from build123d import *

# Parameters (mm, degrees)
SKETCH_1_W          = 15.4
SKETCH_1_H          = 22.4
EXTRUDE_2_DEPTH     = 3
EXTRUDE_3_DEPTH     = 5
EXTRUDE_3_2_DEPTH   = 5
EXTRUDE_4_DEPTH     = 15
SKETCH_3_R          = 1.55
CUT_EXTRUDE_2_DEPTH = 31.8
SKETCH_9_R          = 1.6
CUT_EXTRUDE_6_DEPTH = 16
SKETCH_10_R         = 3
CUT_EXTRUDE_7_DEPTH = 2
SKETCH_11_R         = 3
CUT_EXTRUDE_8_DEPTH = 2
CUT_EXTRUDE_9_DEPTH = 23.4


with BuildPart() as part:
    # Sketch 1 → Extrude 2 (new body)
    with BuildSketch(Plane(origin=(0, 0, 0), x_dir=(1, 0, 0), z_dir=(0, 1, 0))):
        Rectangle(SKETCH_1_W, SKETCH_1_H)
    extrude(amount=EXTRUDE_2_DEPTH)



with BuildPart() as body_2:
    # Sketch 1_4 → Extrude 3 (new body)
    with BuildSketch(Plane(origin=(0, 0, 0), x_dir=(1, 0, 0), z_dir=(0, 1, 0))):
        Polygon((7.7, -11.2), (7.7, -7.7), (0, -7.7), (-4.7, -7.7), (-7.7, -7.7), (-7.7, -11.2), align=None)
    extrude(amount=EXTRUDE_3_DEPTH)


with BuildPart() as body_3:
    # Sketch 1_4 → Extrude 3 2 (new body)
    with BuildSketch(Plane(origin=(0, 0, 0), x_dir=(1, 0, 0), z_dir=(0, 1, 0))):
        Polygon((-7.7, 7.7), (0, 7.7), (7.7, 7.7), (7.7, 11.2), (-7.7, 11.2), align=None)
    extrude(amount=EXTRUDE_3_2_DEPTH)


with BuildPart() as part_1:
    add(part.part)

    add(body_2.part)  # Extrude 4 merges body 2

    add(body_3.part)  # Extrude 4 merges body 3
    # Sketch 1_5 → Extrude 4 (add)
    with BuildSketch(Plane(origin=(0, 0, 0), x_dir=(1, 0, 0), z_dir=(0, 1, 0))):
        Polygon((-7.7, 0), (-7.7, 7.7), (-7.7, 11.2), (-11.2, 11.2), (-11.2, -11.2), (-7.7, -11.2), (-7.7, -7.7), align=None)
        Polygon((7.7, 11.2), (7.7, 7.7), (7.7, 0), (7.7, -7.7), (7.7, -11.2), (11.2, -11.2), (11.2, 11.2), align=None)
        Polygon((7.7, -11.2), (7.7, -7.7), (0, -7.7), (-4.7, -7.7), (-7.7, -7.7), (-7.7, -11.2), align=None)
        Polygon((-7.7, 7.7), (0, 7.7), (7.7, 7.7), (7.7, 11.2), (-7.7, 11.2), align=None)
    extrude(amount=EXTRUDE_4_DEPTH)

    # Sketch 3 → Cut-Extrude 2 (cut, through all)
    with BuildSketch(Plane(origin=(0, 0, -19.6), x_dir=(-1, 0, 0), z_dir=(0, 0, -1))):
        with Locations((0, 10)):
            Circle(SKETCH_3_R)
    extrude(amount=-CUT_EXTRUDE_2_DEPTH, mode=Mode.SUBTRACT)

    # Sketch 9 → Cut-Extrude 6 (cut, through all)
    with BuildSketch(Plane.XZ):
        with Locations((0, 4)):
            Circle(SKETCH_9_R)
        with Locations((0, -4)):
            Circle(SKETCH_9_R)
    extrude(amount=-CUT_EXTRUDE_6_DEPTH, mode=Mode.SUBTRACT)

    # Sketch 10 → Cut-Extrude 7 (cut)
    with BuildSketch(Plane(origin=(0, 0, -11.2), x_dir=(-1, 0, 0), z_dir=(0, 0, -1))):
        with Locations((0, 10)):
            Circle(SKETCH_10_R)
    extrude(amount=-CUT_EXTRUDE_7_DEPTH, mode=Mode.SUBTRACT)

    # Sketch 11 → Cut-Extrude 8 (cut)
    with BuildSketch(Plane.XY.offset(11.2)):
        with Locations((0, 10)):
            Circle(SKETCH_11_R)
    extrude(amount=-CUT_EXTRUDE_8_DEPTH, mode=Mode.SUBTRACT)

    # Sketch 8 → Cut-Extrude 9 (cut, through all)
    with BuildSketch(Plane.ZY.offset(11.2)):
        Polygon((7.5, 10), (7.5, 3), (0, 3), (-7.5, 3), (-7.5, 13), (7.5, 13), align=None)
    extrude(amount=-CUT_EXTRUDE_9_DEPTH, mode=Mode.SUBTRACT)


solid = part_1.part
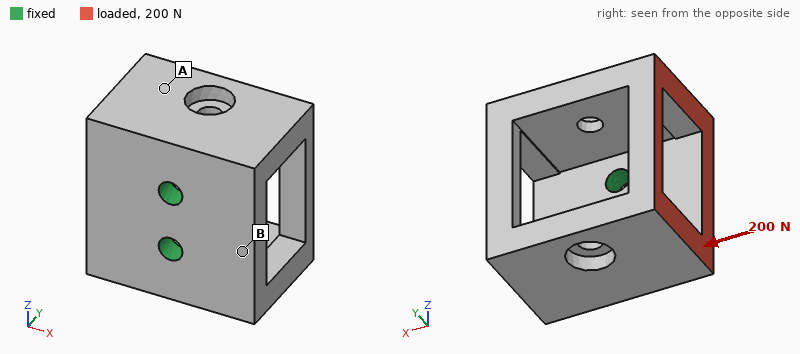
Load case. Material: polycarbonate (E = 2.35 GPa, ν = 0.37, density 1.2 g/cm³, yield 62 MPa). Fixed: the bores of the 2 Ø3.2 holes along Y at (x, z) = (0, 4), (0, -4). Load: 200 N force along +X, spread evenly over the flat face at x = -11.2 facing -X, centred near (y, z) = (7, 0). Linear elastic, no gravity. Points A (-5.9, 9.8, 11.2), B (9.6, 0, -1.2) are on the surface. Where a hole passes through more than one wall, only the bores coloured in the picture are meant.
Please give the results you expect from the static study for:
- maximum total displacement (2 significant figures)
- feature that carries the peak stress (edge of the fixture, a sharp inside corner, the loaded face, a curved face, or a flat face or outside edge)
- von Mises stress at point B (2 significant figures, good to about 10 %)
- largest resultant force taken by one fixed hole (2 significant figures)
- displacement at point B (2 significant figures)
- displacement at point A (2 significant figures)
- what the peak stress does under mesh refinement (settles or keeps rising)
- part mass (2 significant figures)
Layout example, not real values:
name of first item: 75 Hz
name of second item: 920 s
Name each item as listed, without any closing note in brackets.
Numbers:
maximum total displacement: 0.35 mm
feature that carries the peak stress: edge of the fixture
von Mises stress at point B: 5.9 MPa
largest resultant force taken by one fixed hole: 100 N
displacement at point B: 0.10 mm
displacement at point A: 0.16 mm
what the peak stress does under mesh refinement: keeps rising
part mass: 4.1 g
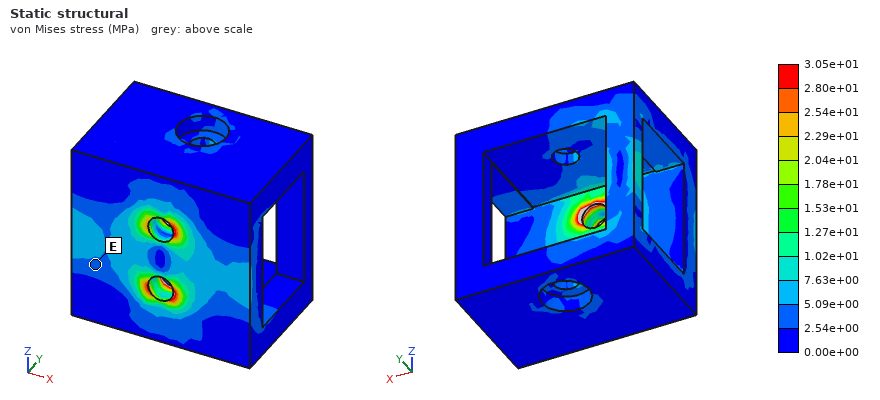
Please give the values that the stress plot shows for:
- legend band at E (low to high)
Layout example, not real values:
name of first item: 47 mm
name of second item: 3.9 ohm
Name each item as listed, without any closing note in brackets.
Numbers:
legend band at E: 2.54e+00 to 5.09e+00 MPa
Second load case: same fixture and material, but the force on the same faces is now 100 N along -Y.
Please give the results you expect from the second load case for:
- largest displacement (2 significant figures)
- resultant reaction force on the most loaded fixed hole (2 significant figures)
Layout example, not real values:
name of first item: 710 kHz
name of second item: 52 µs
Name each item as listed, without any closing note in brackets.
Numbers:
largest displacement: 0.34 mm
resultant reaction force on the most loaded fixed hole: 51 N
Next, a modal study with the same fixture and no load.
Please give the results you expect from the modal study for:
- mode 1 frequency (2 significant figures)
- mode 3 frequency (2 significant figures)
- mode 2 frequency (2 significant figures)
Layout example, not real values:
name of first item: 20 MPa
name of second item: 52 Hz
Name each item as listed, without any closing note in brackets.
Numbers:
mode 1 frequency: 2300 Hz
mode 3 frequency: 3300 Hz
mode 2 frequency: 2300 Hz
